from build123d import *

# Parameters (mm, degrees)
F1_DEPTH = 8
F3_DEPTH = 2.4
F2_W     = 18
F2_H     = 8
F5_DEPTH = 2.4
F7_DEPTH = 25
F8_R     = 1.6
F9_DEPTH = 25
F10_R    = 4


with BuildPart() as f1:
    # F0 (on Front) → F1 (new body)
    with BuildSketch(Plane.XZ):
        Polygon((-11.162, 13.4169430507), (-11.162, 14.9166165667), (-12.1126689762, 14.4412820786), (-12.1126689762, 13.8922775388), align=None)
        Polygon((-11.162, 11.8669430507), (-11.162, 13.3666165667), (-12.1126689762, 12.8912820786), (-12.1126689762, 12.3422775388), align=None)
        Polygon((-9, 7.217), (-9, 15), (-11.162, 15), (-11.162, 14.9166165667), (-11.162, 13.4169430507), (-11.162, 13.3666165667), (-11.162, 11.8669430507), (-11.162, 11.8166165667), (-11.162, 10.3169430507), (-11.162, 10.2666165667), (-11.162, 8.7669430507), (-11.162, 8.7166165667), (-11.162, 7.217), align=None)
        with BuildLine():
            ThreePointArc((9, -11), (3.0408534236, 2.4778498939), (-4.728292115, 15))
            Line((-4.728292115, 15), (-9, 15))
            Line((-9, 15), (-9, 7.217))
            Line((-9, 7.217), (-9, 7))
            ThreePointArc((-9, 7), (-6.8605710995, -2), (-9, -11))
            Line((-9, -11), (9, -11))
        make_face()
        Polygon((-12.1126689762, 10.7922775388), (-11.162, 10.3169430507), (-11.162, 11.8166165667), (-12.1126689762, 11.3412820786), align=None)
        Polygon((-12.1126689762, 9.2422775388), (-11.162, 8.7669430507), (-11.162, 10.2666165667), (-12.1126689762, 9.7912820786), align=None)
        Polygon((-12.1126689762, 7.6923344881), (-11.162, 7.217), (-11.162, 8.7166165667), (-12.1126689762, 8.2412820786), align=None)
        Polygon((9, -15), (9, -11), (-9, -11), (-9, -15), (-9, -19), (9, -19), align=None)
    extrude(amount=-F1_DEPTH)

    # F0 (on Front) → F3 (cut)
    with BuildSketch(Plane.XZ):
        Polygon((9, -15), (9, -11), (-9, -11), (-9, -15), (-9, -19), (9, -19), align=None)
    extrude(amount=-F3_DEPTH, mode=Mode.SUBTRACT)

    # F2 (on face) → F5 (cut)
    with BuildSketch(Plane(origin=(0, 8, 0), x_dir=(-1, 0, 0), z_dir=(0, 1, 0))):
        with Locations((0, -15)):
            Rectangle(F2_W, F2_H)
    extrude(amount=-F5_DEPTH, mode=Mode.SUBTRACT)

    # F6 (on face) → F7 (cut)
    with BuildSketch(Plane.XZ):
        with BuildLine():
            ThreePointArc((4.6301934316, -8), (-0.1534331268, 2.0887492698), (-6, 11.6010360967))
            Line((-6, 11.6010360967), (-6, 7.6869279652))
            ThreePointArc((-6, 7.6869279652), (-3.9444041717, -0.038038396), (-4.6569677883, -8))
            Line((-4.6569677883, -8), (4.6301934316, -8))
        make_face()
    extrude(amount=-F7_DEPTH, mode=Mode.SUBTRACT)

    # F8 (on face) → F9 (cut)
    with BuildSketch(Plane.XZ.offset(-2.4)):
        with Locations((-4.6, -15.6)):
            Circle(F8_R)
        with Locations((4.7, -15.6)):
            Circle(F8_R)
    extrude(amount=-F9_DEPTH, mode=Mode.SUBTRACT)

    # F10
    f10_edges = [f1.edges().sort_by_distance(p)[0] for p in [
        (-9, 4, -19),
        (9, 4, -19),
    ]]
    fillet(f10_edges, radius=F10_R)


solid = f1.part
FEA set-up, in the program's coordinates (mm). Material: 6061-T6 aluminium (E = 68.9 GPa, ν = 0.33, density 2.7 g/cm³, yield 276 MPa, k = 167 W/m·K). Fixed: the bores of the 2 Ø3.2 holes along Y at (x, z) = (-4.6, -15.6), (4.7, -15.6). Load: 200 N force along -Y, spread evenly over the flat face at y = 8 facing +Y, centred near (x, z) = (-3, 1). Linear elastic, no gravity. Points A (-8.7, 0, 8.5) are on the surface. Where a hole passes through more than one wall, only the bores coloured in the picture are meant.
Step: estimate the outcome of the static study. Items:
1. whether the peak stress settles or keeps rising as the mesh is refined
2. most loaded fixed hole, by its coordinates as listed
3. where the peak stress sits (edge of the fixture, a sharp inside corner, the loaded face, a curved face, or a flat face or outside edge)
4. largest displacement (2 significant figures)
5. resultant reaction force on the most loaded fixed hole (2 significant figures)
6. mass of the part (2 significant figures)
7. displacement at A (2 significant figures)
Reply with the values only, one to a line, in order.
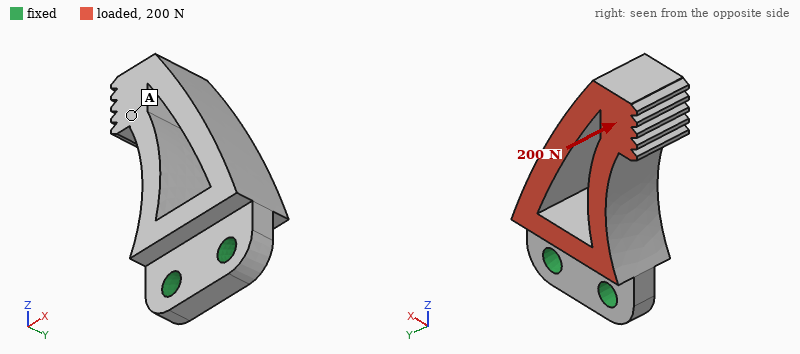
keeps rising
(-4.6, -15.6)
edge of the fixture
0.14 mm
140 N
5.7 g
0.11 mm
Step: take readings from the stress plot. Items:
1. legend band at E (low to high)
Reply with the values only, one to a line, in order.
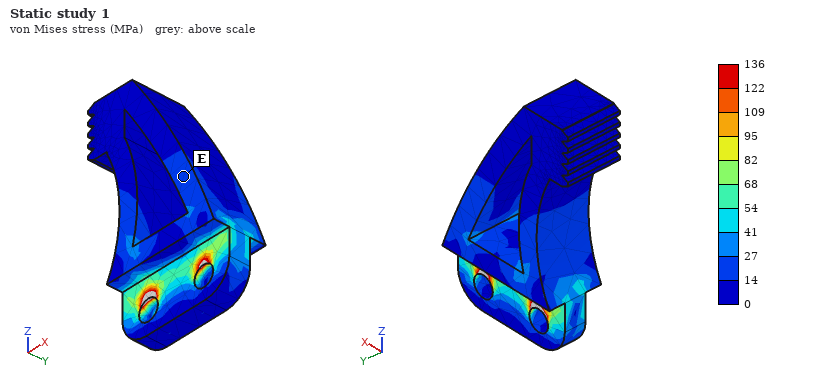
14 to 27 MPa
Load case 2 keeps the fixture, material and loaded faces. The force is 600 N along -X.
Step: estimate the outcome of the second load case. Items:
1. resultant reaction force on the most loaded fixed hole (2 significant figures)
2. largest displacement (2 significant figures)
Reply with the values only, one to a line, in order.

900 N
95 µm
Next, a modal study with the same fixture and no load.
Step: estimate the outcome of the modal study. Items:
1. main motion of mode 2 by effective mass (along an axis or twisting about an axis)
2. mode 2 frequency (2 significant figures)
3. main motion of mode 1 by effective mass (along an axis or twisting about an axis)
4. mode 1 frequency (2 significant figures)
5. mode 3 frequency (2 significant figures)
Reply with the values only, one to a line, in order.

along X
7800 Hz
along Y
3400 Hz
14 kHz
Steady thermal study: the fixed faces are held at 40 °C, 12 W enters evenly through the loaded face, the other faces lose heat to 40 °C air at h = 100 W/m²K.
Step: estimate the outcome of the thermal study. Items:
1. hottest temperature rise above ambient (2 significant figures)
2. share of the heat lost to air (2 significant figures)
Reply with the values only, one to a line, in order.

20 K
15 %
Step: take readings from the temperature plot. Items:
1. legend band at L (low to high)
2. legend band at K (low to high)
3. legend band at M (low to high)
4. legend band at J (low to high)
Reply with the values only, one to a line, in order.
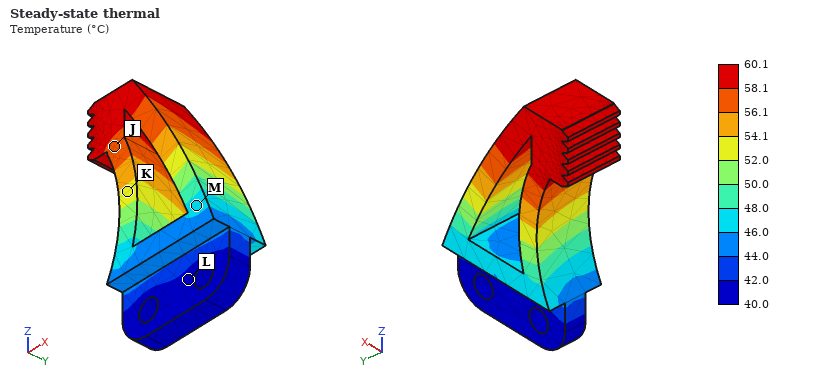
40.0 to 42.0 °C
52.0 to 54.1 °C
46.0 to 48.0 °C
56.1 to 58.1 °C
